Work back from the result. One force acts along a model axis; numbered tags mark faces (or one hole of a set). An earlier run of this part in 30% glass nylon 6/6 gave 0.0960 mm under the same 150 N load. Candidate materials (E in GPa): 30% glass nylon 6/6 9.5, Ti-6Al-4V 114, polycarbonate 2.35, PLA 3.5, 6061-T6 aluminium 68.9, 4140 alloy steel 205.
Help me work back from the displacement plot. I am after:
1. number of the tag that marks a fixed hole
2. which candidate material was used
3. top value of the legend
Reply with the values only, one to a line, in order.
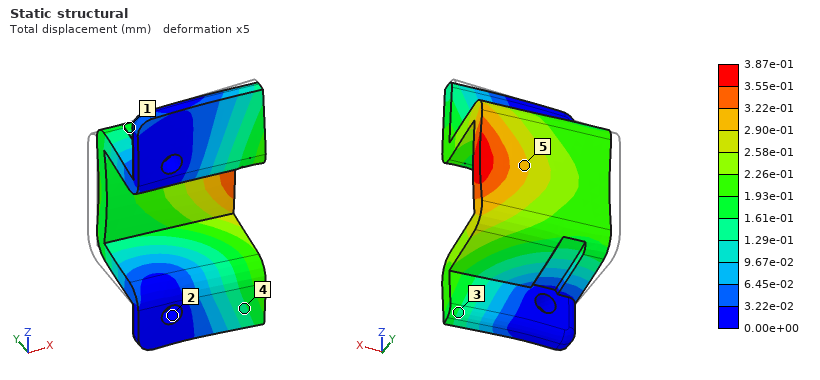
2
polycarbonate
3.87e-01 mm
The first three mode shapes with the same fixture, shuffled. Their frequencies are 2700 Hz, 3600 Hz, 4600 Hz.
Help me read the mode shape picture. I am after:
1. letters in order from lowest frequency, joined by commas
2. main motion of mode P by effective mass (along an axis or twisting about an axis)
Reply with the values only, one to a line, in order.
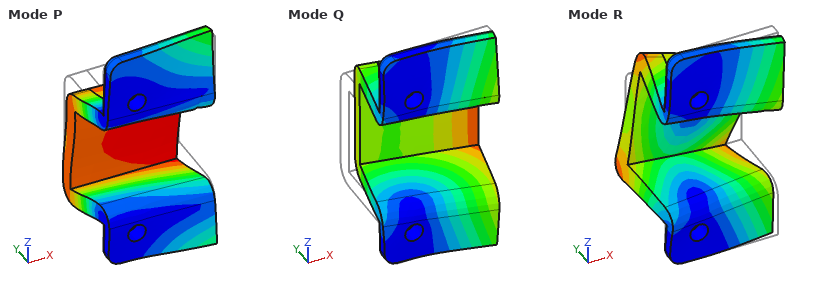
Q, P, R
along Z
